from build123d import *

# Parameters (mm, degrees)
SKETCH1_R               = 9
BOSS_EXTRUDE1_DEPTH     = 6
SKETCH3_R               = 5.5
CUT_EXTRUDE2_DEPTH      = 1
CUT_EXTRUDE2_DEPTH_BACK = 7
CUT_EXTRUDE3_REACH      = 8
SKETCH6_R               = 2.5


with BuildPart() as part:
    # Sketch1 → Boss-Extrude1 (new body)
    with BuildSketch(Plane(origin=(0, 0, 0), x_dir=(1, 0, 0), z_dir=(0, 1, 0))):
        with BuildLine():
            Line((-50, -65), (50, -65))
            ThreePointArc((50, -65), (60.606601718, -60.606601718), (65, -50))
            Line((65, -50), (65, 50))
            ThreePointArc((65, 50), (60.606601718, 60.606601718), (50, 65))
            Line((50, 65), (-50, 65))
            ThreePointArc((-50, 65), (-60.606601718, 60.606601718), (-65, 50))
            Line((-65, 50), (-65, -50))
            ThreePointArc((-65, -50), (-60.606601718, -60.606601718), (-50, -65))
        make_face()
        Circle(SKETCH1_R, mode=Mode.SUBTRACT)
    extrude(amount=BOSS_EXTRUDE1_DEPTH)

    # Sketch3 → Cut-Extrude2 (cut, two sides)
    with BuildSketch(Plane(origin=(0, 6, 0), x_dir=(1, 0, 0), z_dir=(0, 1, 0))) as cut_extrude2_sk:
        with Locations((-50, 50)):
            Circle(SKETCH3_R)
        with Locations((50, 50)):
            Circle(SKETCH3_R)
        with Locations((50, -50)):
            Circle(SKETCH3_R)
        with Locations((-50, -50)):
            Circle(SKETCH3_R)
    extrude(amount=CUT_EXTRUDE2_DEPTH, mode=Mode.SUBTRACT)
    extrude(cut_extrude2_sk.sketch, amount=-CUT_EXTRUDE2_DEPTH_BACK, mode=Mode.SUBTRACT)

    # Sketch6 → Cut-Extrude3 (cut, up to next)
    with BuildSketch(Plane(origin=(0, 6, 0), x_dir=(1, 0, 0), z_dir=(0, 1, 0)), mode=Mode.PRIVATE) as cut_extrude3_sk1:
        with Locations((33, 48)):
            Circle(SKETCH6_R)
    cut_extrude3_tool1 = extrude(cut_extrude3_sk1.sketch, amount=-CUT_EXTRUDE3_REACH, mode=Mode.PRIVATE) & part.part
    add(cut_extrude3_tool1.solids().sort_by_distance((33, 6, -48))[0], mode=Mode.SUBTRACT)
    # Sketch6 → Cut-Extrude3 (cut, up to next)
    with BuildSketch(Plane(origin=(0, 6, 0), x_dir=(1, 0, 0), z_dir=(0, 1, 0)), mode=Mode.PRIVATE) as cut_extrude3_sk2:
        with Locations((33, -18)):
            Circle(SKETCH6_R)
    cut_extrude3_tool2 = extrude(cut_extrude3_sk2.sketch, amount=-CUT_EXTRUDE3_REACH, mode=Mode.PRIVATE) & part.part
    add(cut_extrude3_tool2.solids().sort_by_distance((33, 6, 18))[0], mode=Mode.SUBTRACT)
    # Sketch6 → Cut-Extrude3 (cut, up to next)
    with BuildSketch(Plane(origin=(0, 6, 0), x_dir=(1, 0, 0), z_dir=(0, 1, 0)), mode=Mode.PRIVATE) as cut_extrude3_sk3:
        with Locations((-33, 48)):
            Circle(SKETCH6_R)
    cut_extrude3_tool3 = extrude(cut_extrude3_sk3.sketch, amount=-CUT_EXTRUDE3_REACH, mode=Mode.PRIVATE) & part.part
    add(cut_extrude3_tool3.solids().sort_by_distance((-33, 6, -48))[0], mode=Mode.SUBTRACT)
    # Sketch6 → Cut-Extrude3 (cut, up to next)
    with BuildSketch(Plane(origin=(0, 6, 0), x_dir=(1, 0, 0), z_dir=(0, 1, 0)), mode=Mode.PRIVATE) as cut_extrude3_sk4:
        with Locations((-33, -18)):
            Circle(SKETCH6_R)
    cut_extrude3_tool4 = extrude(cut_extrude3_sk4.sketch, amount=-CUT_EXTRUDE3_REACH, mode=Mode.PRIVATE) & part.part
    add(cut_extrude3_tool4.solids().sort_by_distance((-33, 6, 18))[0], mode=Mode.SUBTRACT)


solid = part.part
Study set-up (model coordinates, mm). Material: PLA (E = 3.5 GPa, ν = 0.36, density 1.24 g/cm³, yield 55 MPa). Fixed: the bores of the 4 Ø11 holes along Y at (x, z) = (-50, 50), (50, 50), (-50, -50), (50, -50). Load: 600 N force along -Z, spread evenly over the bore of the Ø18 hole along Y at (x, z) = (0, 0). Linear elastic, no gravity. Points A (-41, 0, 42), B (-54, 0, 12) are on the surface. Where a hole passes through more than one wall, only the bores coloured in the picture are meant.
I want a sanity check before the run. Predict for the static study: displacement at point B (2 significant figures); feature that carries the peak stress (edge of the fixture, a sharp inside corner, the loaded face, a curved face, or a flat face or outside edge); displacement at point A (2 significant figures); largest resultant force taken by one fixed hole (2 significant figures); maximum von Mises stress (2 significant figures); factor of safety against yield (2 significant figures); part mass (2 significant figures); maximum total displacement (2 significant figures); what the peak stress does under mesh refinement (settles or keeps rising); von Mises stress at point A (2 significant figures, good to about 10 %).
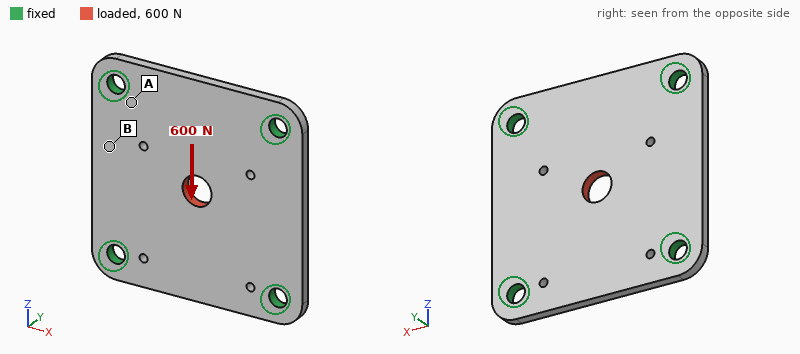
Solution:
4.0 µm
the loaded face
3.6 µm
170 N
3.1 MPa
18
120 g
24 µm
settles
1.2 MPa
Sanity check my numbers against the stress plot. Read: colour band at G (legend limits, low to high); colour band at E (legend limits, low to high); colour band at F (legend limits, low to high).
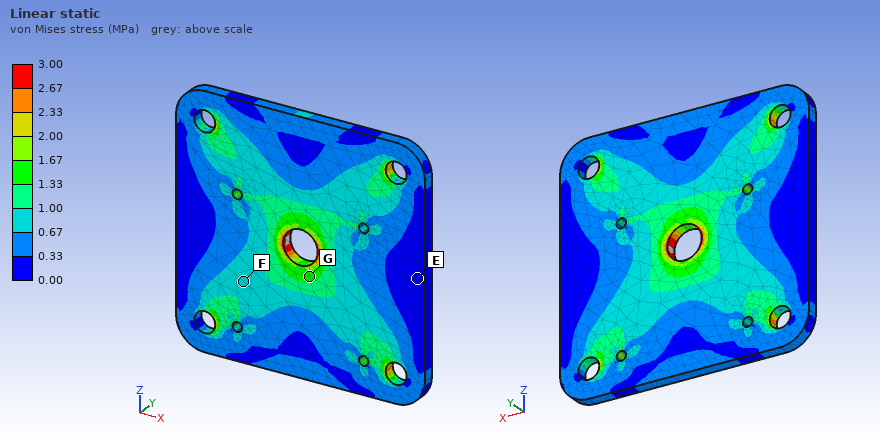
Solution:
1.33 to 1.67 MPa
0.00 to 0.33 MPa
0.67 to 1.00 MPa
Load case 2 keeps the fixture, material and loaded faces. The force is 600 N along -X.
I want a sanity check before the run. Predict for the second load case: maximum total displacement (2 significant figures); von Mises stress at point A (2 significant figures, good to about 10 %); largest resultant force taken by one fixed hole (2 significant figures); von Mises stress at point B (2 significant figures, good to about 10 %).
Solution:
24 µm
1.2 MPa
170 N
0.35 MPa
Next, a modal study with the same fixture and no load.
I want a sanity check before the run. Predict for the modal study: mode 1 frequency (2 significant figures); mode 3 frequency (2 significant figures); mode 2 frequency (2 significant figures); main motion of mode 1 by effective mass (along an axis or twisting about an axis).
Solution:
790 Hz
1200 Hz
1200 Hz
along Y
